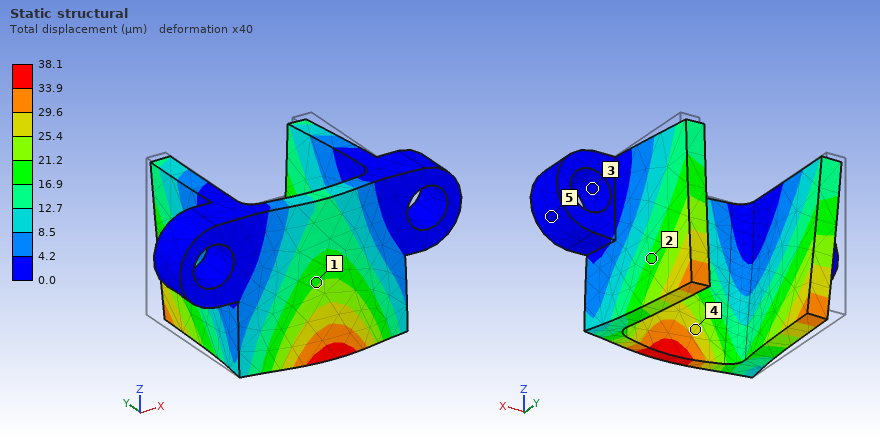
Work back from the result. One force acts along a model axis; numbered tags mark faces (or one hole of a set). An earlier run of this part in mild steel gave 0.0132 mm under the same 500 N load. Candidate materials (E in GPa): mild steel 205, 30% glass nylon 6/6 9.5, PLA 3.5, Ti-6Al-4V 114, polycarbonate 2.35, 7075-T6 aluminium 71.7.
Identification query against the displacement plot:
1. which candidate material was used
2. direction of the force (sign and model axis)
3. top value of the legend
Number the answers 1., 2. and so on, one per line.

1. 7075-T6 aluminium
2. -Y
3. 38.1 µm
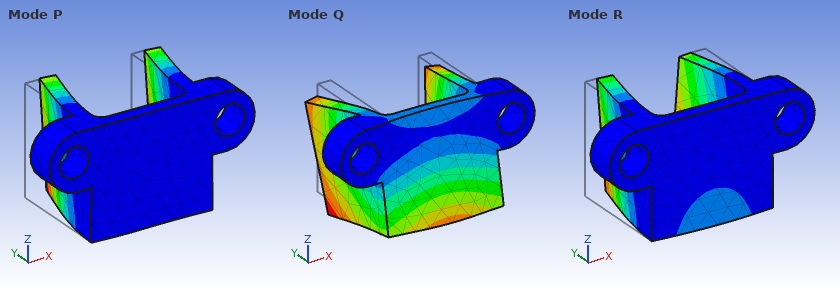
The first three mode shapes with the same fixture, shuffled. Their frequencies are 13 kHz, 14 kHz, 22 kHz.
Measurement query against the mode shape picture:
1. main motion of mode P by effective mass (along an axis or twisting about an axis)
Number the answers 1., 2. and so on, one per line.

1. along X
